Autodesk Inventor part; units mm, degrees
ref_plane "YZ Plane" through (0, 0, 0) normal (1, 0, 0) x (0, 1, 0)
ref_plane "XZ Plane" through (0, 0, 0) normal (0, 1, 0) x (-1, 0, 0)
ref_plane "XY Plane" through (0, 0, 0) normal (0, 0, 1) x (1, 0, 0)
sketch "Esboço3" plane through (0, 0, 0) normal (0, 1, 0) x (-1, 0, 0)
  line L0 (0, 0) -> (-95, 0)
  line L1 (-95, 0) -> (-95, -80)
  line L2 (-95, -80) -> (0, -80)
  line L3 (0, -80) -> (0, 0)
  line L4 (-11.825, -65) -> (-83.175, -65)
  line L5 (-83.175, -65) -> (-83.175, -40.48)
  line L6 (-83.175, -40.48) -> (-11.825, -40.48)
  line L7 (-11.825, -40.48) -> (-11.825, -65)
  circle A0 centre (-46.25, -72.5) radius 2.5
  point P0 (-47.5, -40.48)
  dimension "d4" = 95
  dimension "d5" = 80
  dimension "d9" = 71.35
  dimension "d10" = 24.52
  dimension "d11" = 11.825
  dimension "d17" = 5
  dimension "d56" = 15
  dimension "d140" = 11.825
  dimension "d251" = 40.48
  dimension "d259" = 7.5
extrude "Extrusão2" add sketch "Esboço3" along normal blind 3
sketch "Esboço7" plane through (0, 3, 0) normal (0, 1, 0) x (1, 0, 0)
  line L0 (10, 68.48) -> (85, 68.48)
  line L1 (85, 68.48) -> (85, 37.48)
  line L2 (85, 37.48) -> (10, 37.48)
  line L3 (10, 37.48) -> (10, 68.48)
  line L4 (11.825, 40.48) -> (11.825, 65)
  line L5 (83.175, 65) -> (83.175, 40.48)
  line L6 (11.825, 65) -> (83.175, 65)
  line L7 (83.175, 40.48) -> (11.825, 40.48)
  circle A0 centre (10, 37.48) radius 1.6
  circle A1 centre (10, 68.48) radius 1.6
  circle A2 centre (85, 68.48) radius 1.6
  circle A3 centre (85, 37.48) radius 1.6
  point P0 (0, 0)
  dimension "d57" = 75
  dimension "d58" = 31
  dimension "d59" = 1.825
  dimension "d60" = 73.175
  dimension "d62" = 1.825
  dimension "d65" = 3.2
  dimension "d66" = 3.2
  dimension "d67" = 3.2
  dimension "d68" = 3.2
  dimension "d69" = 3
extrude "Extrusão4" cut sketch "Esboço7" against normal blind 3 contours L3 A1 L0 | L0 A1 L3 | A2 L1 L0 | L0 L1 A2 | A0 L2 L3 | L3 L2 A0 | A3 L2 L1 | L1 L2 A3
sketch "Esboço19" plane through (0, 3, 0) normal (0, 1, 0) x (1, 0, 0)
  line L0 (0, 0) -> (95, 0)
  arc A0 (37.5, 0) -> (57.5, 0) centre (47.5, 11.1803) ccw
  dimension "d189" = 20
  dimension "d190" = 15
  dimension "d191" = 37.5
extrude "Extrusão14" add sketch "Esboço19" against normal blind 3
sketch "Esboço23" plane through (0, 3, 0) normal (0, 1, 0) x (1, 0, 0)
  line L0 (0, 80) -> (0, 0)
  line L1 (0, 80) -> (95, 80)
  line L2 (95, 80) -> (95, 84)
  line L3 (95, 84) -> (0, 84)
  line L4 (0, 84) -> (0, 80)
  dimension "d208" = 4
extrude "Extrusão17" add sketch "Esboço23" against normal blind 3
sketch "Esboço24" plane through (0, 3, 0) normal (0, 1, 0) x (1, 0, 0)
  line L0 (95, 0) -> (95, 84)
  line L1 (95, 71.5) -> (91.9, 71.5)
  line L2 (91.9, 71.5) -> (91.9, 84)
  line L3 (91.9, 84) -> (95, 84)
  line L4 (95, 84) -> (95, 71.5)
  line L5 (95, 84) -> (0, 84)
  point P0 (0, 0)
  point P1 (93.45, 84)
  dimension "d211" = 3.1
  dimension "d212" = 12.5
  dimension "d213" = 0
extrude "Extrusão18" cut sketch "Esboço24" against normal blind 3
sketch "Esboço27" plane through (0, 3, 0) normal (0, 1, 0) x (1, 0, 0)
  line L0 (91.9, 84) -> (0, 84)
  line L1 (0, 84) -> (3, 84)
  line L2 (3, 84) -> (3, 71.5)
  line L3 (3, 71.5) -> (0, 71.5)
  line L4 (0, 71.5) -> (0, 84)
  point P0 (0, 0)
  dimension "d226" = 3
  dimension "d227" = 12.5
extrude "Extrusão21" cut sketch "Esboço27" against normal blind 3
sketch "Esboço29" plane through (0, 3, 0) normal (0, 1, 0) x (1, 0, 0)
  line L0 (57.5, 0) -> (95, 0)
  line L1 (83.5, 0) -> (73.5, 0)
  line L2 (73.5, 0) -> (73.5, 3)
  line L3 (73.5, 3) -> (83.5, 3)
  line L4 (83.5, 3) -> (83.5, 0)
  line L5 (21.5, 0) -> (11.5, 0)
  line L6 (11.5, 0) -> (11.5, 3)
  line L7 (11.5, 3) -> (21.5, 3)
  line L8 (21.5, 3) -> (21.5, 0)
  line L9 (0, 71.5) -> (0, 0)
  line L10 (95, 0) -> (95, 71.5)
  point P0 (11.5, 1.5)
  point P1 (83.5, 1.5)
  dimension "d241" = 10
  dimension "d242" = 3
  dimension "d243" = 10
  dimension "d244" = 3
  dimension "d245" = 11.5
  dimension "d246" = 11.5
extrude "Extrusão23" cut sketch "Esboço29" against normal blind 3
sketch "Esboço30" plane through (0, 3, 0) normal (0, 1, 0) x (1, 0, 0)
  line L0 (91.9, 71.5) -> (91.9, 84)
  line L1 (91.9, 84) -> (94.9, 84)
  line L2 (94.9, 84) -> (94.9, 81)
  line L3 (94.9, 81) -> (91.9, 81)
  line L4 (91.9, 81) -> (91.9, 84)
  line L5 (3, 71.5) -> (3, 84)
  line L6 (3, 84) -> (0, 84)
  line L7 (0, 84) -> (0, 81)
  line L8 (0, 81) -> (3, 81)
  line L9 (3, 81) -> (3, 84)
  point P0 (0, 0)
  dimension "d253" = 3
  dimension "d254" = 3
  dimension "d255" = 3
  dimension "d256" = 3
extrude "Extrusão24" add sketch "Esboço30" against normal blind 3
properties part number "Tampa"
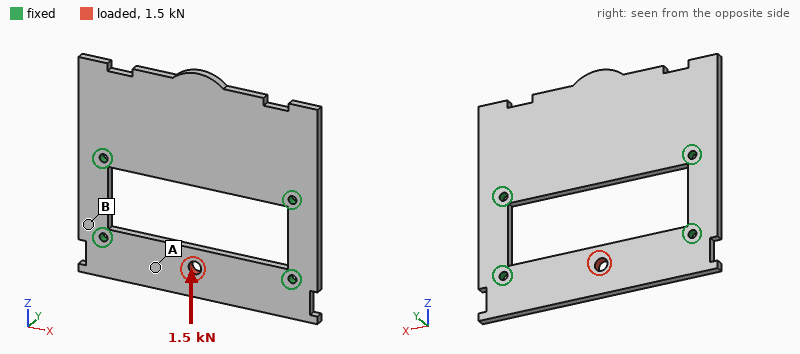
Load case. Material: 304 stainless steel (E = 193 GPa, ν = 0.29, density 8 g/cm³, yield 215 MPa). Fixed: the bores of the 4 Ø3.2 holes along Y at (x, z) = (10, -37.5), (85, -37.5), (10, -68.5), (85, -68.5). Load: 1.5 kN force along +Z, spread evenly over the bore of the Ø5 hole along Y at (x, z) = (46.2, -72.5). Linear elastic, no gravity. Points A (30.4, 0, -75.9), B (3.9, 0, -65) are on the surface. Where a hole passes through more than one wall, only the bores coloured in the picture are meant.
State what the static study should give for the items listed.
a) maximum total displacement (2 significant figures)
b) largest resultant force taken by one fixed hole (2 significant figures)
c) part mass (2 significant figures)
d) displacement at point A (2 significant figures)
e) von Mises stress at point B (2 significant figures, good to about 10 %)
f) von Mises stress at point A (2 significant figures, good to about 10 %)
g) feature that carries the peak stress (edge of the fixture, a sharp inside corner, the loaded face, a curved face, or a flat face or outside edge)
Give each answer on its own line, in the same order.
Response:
26 µm
1.2 kN
150 g
17 µm
14 MPa
40 MPa
edge of the fixture
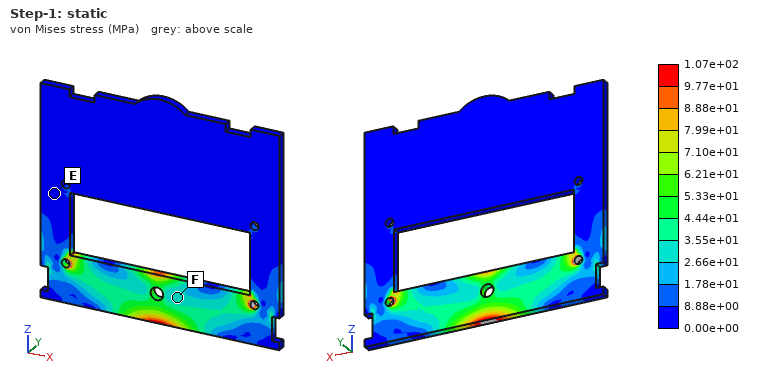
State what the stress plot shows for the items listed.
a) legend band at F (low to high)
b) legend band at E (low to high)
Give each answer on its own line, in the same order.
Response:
2.66e+01 to 3.55e+01 MPa
0.00e+00 to 8.88e+00 MPa
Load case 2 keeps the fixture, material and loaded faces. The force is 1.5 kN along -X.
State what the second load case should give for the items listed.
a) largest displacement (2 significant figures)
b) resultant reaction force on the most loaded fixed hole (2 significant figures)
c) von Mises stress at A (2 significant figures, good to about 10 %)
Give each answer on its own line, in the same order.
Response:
4.2 µm
790 N
13 MPa
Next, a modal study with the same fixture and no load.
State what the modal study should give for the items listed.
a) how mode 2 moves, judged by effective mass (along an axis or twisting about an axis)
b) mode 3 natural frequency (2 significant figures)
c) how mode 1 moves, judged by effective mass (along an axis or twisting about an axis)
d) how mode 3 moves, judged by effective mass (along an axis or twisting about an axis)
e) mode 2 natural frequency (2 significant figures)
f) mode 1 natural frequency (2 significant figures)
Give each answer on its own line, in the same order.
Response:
twisting about Z
2400 Hz
along Y
along Y
2200 Hz
1100 Hz
